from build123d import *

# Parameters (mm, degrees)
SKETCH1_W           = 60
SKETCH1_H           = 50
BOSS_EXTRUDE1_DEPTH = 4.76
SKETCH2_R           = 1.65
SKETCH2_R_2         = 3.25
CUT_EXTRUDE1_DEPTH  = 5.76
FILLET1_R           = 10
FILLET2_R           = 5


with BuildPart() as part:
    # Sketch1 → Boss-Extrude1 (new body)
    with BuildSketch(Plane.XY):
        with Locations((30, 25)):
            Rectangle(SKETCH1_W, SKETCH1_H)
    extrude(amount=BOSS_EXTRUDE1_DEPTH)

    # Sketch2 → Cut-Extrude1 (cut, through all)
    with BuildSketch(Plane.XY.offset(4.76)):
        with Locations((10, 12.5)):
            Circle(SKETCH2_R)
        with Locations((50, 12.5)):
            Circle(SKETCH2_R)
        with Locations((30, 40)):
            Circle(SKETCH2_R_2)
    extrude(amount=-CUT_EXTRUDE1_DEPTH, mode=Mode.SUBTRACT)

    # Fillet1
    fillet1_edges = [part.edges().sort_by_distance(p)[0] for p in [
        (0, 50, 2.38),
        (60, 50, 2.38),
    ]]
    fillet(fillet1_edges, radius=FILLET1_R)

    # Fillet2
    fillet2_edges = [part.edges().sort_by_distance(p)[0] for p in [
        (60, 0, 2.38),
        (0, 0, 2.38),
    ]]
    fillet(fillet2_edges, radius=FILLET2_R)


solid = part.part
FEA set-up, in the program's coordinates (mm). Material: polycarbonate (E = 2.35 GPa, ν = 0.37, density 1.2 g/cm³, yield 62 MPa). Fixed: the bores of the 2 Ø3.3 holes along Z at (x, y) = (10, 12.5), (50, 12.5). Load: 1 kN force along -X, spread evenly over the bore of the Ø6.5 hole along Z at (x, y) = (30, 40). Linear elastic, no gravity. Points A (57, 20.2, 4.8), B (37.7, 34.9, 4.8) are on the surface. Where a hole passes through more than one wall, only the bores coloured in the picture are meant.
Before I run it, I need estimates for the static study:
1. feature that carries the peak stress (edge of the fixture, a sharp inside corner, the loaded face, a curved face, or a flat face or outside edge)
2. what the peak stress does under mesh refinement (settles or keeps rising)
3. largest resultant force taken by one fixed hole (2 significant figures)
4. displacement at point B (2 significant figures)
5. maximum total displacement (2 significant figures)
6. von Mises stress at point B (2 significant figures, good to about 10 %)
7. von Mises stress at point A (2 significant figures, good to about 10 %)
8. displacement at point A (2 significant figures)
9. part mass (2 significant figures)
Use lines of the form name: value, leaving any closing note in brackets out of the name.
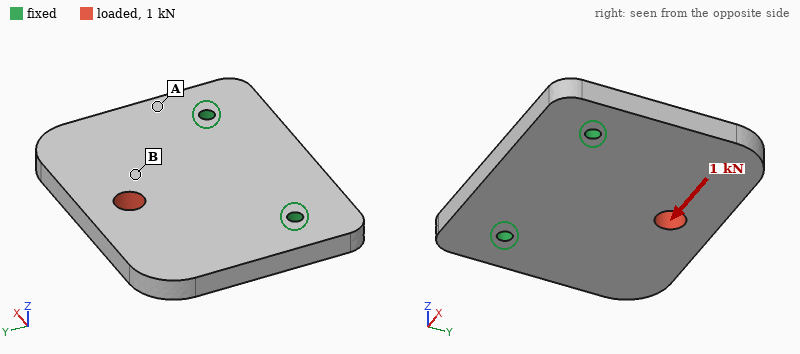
feature that carries the peak stress: edge of the fixture
what the peak stress does under mesh refinement: keeps rising
largest resultant force taken by one fixed hole: 830 N
displacement at point B: 0.17 mm
maximum total displacement: 0.26 mm
von Mises stress at point B: 9.1 MPa
von Mises stress at point A: 4.8 MPa
displacement at point A: 0.093 mm
part mass: 17 g
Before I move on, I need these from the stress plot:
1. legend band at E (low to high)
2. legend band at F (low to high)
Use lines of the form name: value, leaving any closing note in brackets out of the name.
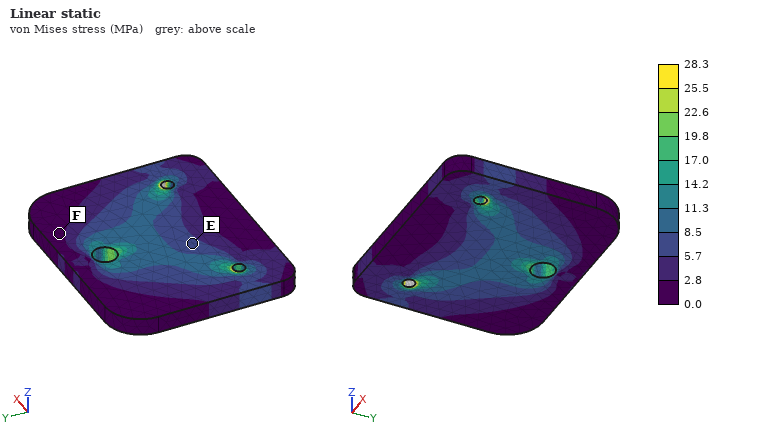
legend band at E: 5.7 to 8.5 MPa
legend band at F: 0.0 to 2.8 MPa
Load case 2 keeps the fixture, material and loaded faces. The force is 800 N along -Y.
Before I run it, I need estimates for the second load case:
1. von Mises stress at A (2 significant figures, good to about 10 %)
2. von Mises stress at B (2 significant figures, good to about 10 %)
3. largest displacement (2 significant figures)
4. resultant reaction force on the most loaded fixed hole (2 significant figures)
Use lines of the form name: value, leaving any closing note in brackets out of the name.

von Mises stress at A: 1.5 MPa
von Mises stress at B: 5.7 MPa
largest displacement: 0.12 mm
resultant reaction force on the most loaded fixed hole: 420 N
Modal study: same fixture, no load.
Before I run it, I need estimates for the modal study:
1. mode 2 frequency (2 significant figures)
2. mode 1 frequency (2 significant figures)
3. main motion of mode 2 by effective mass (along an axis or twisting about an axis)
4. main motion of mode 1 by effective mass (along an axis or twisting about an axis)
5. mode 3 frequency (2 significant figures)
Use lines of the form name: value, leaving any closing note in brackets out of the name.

mode 2 frequency: 1300 Hz
mode 1 frequency: 680 Hz
main motion of mode 2 by effective mass: twisting about Y
main motion of mode 1 by effective mass: along Z
mode 3 frequency: 2600 Hz
